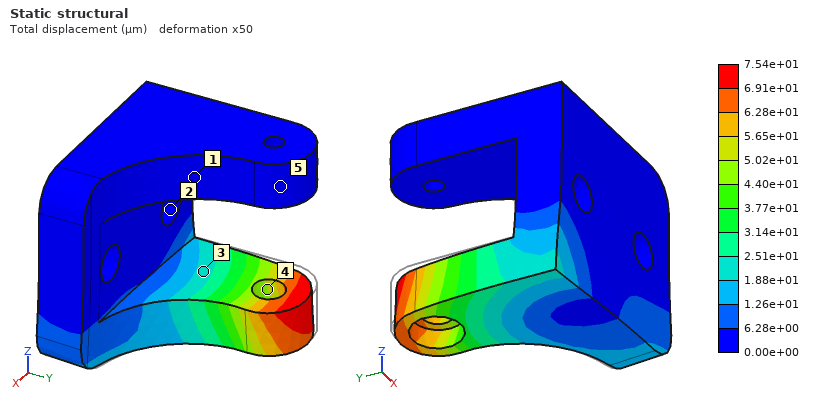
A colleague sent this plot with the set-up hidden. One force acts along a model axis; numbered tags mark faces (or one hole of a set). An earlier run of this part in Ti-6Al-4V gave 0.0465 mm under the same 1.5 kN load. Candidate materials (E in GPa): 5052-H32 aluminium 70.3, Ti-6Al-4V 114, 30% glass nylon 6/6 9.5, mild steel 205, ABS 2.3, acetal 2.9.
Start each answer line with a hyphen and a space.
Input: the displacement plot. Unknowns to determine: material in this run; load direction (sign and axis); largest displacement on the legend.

- 5052-H32 aluminium
- +X
- 7.54e+01 µm
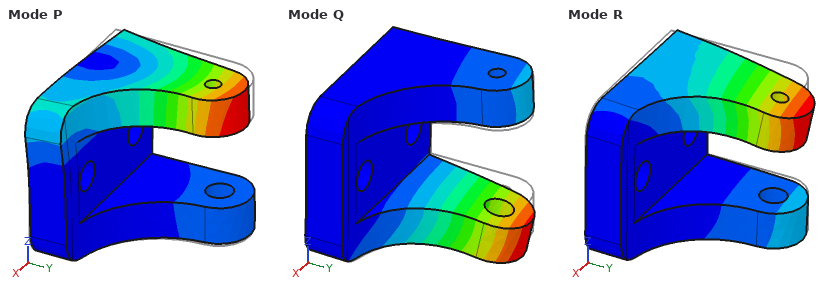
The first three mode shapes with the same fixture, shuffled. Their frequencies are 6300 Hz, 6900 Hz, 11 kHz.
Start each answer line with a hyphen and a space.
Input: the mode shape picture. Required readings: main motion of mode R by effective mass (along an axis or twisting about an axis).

- along Z
